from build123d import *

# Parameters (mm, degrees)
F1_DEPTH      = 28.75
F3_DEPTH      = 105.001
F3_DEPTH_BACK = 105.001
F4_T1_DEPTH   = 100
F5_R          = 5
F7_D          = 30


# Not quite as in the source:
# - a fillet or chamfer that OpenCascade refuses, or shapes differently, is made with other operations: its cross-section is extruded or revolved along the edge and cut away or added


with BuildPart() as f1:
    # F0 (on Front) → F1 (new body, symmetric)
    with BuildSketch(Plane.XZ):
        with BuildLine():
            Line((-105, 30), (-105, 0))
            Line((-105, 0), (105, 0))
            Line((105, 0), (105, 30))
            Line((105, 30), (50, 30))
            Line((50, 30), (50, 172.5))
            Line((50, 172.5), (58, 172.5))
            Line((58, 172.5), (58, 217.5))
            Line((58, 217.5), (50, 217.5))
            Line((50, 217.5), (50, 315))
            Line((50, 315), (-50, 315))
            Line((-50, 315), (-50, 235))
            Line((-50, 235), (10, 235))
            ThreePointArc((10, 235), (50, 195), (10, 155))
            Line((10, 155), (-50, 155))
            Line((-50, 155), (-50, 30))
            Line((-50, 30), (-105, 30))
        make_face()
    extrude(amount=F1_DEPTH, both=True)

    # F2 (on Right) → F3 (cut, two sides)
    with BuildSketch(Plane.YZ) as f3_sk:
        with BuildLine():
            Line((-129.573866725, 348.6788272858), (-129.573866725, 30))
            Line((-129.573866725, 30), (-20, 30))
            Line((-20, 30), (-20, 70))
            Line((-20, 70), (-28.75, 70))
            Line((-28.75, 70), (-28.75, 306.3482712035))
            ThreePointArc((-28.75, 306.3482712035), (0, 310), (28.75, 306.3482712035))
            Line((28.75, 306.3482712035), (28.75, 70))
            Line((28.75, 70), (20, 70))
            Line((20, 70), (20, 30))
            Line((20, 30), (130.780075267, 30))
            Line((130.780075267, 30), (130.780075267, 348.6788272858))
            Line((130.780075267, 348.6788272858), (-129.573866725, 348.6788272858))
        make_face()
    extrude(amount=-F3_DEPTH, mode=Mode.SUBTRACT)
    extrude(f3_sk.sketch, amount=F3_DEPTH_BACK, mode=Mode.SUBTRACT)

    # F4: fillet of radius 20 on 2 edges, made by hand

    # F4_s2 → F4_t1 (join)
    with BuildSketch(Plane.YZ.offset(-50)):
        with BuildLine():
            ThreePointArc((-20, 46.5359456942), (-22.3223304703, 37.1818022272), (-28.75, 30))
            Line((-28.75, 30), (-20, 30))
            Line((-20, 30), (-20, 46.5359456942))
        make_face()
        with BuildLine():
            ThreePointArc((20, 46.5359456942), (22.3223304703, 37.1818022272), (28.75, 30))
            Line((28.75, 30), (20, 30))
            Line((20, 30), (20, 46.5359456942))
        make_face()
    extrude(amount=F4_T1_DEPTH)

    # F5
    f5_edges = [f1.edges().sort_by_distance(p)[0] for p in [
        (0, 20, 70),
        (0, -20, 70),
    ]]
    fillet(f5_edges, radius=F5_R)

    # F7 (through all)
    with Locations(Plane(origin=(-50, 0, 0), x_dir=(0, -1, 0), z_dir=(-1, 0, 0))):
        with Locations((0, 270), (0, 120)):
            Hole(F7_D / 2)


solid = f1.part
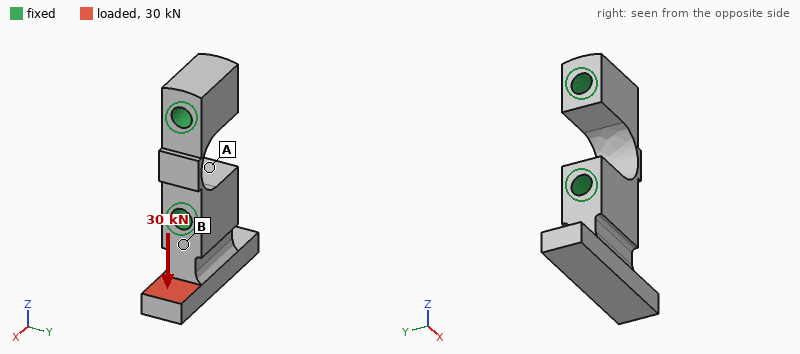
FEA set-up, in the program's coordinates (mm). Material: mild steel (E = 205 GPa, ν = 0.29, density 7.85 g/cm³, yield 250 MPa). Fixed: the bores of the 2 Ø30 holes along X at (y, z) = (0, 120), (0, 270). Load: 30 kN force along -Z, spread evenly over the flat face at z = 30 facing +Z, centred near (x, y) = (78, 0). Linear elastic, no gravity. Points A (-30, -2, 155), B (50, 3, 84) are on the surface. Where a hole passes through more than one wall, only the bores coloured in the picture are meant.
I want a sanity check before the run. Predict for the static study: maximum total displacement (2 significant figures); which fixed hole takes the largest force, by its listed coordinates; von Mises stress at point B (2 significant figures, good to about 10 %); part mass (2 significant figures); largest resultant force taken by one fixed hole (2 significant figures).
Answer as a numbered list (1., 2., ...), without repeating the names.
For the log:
1. 0.11 mm
2. (0, 120)
3. 40 MPa
4. 11 kg
5. 30 kN
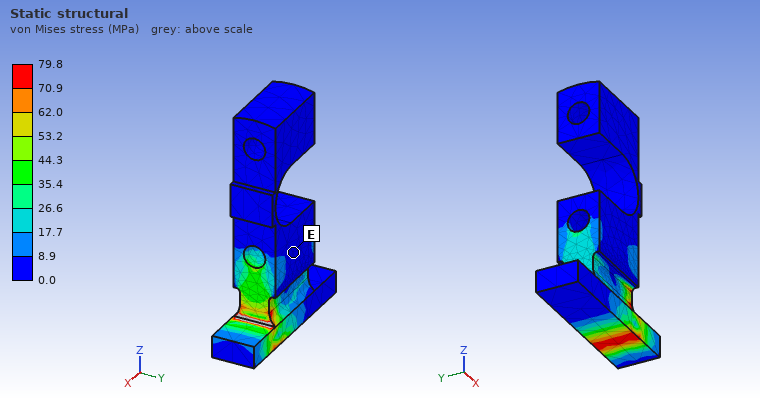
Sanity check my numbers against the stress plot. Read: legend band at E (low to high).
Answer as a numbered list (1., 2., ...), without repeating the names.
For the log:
1. 0.0 to 8.9 MPa
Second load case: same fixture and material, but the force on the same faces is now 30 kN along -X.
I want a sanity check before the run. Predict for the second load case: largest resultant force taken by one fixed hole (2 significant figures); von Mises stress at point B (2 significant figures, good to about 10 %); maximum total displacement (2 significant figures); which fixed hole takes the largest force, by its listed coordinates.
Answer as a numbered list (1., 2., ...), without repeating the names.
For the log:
1. 30 kN
2. 27 MPa
3. 33 µm
4. (0, 120)
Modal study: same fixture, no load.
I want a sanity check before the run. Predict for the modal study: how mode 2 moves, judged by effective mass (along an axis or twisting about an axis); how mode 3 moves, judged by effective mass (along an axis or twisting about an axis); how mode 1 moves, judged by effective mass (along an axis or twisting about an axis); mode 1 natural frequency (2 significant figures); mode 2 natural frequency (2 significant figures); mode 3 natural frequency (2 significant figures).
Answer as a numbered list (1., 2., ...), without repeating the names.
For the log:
1. twisting about Z
2. along X
3. along Y
4. 1900 Hz
5. 2200 Hz
6. 2700 Hz
